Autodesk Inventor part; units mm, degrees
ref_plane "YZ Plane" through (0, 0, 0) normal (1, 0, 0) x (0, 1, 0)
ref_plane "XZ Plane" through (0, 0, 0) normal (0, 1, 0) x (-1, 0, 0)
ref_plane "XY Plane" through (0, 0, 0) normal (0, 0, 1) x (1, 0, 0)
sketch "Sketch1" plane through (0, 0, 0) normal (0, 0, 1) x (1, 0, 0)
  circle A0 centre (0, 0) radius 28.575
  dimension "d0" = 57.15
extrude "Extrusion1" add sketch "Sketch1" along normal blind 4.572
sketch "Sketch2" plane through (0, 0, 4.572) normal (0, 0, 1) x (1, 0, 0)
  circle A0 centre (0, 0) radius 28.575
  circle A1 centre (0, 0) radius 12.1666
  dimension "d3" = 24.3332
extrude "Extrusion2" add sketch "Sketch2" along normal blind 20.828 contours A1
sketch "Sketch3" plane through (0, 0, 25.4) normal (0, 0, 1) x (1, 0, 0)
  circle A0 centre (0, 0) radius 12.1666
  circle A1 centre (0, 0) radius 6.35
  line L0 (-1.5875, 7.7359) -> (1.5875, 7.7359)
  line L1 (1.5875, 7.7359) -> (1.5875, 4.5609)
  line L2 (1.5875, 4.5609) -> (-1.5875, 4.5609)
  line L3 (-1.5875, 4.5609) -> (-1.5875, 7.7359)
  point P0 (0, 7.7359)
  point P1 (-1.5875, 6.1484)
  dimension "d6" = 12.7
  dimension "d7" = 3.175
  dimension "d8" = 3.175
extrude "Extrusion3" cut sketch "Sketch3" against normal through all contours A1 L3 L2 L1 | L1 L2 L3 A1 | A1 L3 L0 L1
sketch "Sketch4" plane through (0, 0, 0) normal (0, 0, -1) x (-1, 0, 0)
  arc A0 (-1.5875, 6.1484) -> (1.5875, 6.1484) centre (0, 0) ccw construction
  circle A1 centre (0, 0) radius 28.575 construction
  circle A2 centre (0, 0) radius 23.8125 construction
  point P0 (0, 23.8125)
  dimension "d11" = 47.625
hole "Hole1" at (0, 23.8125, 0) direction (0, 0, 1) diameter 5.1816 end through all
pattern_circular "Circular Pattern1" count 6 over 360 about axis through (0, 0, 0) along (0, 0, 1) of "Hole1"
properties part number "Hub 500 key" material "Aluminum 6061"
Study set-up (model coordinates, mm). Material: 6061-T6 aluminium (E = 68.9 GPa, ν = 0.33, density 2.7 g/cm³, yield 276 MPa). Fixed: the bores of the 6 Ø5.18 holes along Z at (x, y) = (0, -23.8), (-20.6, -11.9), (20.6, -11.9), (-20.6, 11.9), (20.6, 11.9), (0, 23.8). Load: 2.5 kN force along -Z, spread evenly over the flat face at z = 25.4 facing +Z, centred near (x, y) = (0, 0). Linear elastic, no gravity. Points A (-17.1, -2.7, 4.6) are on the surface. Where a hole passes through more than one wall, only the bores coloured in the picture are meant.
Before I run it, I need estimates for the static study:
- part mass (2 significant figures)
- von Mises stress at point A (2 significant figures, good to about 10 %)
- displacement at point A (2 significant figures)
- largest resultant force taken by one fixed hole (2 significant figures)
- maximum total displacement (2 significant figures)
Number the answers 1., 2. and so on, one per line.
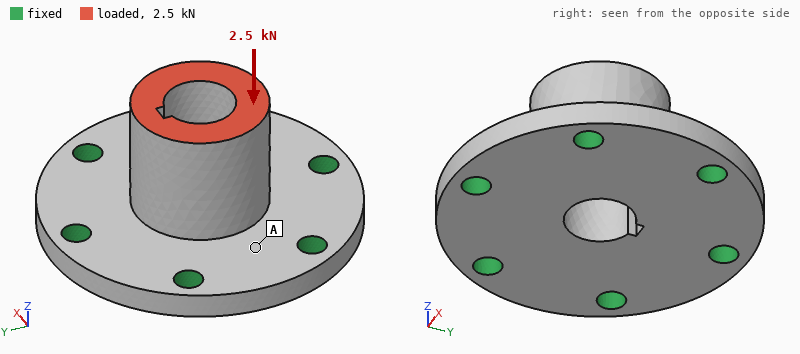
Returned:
1. 47 g
2. 11 MPa
3. 5.8 µm
4. 460 N
5. 15 µm
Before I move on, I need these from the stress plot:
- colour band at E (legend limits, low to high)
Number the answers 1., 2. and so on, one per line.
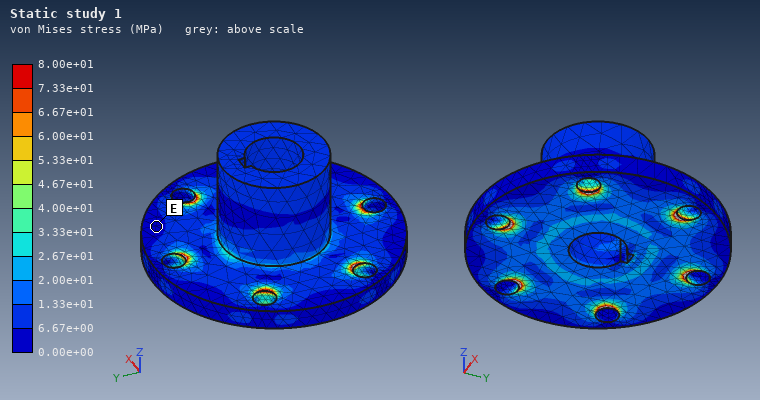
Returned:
1. 0.00e+00 to 6.67e+00 MPa
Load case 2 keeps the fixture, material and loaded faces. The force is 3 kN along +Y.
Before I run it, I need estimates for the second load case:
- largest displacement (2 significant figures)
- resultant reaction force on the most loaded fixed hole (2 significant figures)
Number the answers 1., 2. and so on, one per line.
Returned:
1. 79 µm
2. 1.5 kN
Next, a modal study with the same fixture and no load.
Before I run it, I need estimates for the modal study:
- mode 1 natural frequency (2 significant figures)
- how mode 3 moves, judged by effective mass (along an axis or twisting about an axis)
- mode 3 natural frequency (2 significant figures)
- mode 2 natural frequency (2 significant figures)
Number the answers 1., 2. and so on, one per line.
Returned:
1. 12 kHz
2. along Z
3. 14 kHz
4. 12 kHz
